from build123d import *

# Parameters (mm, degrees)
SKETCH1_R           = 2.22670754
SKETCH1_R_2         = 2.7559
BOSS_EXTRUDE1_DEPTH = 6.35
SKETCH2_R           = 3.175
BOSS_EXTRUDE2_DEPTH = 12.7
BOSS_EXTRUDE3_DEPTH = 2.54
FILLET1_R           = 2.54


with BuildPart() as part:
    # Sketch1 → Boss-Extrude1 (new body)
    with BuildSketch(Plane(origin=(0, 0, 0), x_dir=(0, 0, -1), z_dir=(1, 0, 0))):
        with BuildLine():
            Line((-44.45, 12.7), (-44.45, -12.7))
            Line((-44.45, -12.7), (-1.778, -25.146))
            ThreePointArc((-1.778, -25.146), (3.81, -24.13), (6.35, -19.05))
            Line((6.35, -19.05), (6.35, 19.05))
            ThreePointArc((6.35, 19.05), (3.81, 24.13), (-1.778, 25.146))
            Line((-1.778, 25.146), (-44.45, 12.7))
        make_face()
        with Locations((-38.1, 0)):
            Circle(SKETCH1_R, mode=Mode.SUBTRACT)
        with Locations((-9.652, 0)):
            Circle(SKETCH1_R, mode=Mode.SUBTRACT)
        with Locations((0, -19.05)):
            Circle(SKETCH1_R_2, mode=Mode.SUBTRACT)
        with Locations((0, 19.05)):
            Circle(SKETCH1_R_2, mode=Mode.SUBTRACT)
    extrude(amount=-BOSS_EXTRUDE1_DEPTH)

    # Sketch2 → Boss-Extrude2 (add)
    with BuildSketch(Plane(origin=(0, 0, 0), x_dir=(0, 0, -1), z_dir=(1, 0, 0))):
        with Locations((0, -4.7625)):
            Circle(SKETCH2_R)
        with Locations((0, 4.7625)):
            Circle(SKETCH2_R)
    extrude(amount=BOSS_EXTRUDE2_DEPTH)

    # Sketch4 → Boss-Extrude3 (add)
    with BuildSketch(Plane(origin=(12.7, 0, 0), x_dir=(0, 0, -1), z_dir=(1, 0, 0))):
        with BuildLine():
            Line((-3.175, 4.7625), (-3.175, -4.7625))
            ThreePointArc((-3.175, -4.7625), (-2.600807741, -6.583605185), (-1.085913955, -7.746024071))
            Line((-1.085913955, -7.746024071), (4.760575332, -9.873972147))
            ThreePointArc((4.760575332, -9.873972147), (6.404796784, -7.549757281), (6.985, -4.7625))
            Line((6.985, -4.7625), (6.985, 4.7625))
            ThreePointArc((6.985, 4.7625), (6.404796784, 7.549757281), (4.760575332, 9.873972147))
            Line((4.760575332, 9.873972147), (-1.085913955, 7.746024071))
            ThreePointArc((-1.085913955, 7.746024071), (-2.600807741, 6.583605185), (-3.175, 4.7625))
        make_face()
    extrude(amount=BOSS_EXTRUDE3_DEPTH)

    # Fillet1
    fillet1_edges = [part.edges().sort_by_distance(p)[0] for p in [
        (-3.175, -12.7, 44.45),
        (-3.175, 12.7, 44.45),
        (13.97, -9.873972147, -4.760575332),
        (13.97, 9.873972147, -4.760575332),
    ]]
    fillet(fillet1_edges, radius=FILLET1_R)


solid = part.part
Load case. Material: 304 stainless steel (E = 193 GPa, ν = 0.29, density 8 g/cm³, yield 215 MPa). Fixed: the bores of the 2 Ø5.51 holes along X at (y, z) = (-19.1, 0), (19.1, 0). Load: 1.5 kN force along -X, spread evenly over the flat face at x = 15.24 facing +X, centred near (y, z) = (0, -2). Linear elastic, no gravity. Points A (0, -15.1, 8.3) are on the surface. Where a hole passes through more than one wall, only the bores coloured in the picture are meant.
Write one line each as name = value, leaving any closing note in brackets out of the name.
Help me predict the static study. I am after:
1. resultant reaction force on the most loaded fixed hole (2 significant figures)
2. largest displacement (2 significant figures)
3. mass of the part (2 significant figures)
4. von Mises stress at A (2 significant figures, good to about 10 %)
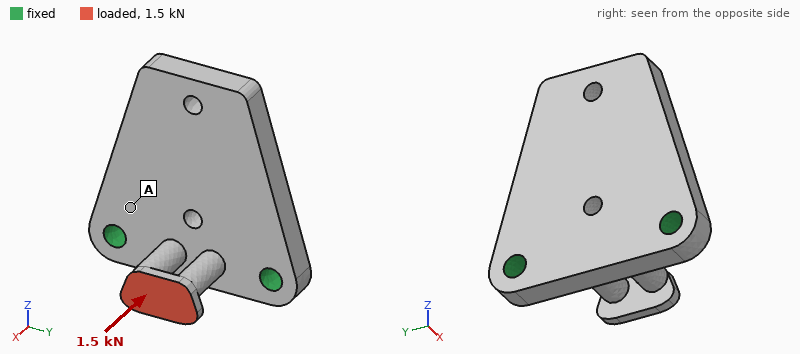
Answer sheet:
resultant reaction force on the most loaded fixed hole = 760 N
largest displacement = 31 µm
mass of the part = 110 g
von Mises stress at A = 11 MPa
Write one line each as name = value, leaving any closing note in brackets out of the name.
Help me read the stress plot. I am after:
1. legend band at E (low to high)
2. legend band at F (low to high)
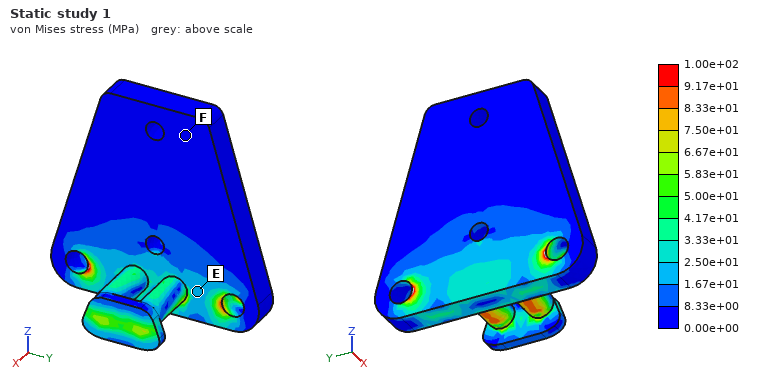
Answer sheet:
legend band at E = 1.67e+01 to 2.50e+01 MPa
legend band at F = 0.00e+00 to 8.33e+00 MPa
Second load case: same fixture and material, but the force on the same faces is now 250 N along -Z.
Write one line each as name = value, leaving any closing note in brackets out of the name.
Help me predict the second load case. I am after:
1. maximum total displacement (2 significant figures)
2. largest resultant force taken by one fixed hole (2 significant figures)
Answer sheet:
maximum total displacement = 21 µm
largest resultant force taken by one fixed hole = 130 N
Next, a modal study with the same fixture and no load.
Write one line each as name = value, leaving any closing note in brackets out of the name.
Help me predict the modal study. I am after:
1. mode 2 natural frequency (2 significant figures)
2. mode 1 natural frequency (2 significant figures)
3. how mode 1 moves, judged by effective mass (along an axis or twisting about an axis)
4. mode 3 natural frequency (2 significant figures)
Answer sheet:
mode 2 natural frequency = 9100 Hz
mode 1 natural frequency = 2800 Hz
how mode 1 moves, judged by effective mass = along X
mode 3 natural frequency = 9200 Hz
